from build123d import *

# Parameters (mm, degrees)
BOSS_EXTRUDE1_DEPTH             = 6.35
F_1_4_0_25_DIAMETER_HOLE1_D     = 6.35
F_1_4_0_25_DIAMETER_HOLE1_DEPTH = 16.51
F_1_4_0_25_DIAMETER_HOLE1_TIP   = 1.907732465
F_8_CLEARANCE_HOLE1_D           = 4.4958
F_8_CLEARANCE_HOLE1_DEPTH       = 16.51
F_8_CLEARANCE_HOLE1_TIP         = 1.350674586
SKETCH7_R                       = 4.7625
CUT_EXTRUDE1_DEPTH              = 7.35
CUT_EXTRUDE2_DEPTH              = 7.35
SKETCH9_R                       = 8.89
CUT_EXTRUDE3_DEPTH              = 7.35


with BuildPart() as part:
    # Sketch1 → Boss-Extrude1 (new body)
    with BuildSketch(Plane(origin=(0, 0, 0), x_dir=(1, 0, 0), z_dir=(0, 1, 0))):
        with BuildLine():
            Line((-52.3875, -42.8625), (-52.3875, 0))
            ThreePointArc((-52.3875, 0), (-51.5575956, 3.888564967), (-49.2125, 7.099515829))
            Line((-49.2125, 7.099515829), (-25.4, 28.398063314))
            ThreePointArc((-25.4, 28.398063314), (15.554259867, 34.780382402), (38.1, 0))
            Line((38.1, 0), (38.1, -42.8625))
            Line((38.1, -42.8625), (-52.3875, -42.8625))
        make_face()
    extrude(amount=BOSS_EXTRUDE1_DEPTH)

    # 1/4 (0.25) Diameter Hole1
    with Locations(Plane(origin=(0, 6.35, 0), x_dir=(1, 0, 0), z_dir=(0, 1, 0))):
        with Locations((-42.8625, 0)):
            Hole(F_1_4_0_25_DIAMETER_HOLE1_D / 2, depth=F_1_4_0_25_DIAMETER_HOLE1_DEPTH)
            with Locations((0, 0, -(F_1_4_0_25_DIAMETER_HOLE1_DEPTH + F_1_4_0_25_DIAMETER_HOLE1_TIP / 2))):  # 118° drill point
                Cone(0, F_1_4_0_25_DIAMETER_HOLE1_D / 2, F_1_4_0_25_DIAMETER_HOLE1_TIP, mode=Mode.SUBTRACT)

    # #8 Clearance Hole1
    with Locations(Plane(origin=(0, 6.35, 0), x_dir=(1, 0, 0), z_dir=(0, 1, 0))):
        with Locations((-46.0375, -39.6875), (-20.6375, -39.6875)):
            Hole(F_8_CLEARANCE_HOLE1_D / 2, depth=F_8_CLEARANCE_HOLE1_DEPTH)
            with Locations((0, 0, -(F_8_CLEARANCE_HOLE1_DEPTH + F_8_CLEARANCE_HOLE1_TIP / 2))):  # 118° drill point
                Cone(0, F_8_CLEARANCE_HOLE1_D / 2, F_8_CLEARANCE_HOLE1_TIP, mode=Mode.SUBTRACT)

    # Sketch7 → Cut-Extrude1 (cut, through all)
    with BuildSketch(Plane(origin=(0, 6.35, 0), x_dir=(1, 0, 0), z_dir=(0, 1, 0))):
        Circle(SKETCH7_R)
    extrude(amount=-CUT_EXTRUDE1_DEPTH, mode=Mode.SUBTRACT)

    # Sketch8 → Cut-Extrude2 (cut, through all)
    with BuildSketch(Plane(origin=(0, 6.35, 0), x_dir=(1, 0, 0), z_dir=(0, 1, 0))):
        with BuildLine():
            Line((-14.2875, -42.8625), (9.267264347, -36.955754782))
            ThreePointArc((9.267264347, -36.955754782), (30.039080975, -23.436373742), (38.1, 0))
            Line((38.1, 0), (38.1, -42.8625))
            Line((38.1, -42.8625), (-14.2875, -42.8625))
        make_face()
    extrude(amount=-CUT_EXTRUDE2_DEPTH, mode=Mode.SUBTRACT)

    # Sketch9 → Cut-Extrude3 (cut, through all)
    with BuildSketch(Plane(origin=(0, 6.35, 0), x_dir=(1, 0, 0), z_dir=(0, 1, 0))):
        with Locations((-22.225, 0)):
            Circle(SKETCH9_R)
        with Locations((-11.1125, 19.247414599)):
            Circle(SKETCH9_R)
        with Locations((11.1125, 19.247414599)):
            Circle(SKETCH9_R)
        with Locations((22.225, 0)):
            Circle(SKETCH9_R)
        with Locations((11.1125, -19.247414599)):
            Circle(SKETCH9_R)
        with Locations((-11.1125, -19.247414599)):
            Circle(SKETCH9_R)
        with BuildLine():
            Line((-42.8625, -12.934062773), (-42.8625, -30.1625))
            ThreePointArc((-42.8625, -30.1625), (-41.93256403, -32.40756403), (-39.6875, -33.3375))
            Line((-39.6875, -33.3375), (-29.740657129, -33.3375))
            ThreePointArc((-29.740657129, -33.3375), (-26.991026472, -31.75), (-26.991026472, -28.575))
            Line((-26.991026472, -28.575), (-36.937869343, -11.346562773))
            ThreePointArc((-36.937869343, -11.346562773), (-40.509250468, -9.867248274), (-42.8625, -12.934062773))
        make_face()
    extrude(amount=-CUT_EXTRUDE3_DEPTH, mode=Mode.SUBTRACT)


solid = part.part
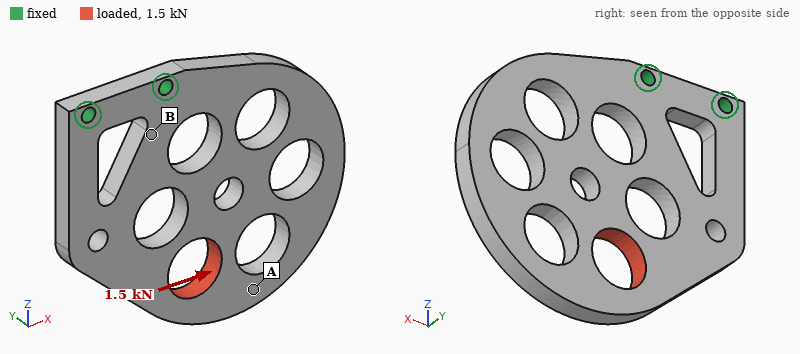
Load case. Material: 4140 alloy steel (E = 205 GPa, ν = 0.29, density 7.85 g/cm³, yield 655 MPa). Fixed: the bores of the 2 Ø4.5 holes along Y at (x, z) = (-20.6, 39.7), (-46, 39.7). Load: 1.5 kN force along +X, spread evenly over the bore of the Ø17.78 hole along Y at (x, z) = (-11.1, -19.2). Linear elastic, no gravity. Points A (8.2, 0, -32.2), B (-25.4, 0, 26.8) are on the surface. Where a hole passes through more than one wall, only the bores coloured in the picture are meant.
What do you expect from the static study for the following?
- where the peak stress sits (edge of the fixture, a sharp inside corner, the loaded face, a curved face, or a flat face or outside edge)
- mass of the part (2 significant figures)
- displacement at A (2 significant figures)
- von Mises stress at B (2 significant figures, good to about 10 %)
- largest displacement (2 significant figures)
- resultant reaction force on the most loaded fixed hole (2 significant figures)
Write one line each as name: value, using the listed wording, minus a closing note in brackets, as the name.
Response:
where the peak stress sits: edge of the fixture
mass of the part: 200 g
displacement at A: 54 µm
von Mises stress at B: 28 MPa
largest displacement: 58 µm
resultant reaction force on the most loaded fixed hole: 2.9 kN
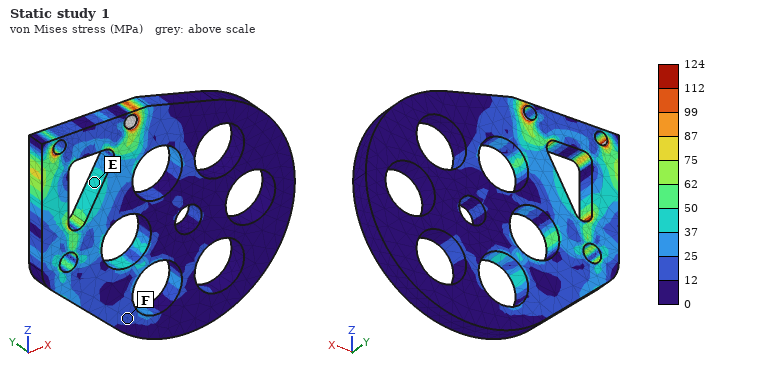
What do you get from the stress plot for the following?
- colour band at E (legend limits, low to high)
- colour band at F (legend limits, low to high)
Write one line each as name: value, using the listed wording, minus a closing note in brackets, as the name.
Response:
colour band at E: 37 to 50 MPa
colour band at F: 12 to 25 MPa
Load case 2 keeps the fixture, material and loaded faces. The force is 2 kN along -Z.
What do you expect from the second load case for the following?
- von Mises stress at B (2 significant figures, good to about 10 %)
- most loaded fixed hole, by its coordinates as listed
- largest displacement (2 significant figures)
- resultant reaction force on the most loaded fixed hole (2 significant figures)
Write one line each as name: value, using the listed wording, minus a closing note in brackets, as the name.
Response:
von Mises stress at B: 30 MPa
most loaded fixed hole, by its coordinates as listed: (-20.6, 39.7)
largest displacement: 29 µm
resultant reaction force on the most loaded fixed hole: 2.5 kN
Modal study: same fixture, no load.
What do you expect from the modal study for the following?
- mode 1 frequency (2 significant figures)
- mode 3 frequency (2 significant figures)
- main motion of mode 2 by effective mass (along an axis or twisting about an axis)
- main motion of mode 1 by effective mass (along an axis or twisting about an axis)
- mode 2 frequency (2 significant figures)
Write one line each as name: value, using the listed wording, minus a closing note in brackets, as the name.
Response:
mode 1 frequency: 630 Hz
mode 3 frequency: 2500 Hz
main motion of mode 2 by effective mass: twisting about Z
main motion of mode 1 by effective mass: along Y
mode 2 frequency: 1400 Hz
